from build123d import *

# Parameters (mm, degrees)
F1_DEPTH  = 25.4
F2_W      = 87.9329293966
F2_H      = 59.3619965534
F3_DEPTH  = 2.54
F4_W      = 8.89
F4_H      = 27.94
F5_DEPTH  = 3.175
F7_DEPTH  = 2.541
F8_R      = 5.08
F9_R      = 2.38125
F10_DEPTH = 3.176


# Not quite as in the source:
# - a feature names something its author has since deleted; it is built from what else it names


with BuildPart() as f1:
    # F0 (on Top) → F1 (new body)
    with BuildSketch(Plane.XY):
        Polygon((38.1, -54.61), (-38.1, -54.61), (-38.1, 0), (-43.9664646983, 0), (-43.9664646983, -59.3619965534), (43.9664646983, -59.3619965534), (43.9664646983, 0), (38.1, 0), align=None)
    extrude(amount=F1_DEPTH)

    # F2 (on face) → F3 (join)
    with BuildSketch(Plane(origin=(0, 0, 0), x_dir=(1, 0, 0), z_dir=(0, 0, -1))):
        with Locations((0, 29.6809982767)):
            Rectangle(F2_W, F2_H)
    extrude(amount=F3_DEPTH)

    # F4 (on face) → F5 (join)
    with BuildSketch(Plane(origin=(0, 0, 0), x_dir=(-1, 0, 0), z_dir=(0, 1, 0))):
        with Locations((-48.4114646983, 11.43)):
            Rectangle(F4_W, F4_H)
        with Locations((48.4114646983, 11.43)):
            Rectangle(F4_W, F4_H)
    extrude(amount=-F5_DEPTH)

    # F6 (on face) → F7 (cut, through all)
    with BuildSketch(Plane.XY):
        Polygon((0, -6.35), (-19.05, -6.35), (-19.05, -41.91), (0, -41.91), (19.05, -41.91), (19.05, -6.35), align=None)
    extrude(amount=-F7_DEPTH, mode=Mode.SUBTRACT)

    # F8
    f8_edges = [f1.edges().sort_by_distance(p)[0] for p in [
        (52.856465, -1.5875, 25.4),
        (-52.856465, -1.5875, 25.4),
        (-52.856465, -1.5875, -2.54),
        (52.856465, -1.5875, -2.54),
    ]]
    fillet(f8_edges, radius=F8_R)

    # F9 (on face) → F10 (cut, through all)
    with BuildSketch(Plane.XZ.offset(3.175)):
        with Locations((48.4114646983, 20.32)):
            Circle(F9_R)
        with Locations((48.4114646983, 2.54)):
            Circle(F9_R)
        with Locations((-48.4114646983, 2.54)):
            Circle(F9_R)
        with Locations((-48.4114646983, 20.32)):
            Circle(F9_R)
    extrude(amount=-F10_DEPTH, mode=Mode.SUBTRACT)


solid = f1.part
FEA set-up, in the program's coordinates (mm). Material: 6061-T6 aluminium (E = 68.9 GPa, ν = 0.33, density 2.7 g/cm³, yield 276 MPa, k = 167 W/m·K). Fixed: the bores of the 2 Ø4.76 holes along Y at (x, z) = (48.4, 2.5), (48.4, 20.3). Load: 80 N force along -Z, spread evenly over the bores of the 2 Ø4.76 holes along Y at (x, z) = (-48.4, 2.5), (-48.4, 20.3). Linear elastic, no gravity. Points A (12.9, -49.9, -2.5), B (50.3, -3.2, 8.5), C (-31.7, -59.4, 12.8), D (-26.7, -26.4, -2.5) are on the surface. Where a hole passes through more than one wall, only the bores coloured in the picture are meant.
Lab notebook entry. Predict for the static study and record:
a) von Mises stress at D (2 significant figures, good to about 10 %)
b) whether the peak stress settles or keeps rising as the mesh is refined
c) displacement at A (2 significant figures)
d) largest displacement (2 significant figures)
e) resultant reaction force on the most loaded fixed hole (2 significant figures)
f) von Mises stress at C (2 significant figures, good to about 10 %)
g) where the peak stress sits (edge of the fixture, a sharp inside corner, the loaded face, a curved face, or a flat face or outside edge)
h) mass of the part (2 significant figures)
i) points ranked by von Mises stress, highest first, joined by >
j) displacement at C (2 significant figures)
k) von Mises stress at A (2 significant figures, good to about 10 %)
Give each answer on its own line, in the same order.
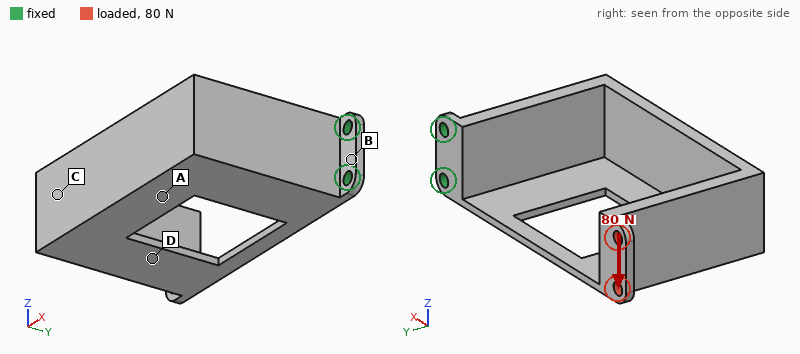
9.9 MPa
keeps rising
0.22 mm
1.2 mm
390 N
16 MPa
a sharp inside corner
100 g
A > C > D > B
0.49 mm
26 MPa
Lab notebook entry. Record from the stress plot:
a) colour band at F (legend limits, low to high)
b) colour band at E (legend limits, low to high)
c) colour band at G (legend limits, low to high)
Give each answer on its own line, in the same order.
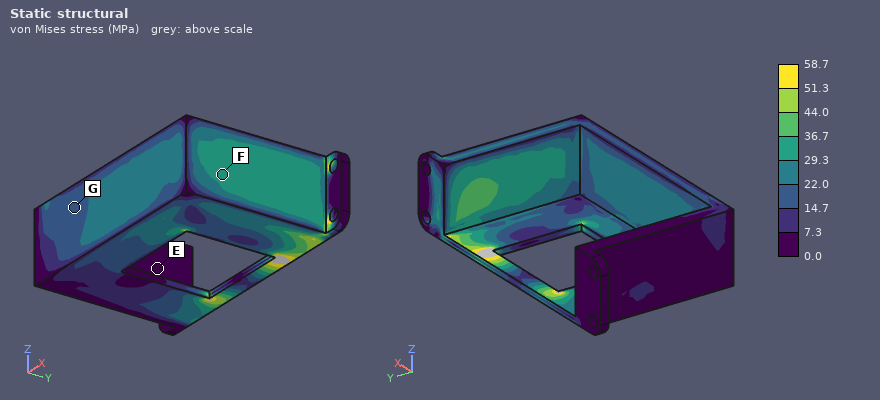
29.3 to 36.7 MPa
0.0 to 7.3 MPa
14.7 to 22.0 MPa
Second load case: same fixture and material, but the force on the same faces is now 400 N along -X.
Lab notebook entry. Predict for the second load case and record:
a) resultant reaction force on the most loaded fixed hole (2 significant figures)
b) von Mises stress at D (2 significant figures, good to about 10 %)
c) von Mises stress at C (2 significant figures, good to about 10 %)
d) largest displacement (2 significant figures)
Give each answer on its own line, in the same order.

200 N
12 MPa
8.8 MPa
0.68 mm
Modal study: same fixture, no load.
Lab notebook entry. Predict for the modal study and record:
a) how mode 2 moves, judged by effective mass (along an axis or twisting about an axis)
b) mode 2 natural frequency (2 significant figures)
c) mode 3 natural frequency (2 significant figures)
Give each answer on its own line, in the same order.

along Z
270 Hz
760 Hz
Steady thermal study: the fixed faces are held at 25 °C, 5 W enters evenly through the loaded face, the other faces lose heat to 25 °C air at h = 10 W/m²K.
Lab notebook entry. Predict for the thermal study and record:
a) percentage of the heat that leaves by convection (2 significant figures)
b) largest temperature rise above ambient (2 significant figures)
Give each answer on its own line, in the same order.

37 %
22 K
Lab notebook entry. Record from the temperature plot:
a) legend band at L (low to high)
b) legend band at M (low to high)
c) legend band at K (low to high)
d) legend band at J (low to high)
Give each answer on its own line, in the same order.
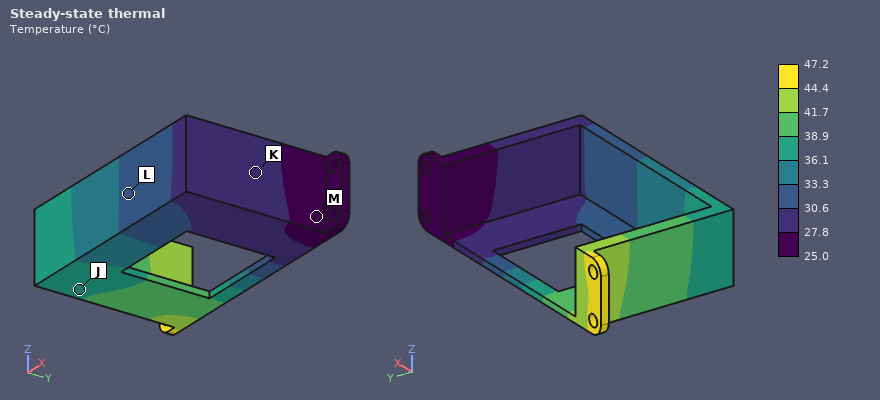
30.6 to 33.3 °C
25.0 to 27.8 °C
27.8 to 30.6 °C
36.1 to 38.9 °C
